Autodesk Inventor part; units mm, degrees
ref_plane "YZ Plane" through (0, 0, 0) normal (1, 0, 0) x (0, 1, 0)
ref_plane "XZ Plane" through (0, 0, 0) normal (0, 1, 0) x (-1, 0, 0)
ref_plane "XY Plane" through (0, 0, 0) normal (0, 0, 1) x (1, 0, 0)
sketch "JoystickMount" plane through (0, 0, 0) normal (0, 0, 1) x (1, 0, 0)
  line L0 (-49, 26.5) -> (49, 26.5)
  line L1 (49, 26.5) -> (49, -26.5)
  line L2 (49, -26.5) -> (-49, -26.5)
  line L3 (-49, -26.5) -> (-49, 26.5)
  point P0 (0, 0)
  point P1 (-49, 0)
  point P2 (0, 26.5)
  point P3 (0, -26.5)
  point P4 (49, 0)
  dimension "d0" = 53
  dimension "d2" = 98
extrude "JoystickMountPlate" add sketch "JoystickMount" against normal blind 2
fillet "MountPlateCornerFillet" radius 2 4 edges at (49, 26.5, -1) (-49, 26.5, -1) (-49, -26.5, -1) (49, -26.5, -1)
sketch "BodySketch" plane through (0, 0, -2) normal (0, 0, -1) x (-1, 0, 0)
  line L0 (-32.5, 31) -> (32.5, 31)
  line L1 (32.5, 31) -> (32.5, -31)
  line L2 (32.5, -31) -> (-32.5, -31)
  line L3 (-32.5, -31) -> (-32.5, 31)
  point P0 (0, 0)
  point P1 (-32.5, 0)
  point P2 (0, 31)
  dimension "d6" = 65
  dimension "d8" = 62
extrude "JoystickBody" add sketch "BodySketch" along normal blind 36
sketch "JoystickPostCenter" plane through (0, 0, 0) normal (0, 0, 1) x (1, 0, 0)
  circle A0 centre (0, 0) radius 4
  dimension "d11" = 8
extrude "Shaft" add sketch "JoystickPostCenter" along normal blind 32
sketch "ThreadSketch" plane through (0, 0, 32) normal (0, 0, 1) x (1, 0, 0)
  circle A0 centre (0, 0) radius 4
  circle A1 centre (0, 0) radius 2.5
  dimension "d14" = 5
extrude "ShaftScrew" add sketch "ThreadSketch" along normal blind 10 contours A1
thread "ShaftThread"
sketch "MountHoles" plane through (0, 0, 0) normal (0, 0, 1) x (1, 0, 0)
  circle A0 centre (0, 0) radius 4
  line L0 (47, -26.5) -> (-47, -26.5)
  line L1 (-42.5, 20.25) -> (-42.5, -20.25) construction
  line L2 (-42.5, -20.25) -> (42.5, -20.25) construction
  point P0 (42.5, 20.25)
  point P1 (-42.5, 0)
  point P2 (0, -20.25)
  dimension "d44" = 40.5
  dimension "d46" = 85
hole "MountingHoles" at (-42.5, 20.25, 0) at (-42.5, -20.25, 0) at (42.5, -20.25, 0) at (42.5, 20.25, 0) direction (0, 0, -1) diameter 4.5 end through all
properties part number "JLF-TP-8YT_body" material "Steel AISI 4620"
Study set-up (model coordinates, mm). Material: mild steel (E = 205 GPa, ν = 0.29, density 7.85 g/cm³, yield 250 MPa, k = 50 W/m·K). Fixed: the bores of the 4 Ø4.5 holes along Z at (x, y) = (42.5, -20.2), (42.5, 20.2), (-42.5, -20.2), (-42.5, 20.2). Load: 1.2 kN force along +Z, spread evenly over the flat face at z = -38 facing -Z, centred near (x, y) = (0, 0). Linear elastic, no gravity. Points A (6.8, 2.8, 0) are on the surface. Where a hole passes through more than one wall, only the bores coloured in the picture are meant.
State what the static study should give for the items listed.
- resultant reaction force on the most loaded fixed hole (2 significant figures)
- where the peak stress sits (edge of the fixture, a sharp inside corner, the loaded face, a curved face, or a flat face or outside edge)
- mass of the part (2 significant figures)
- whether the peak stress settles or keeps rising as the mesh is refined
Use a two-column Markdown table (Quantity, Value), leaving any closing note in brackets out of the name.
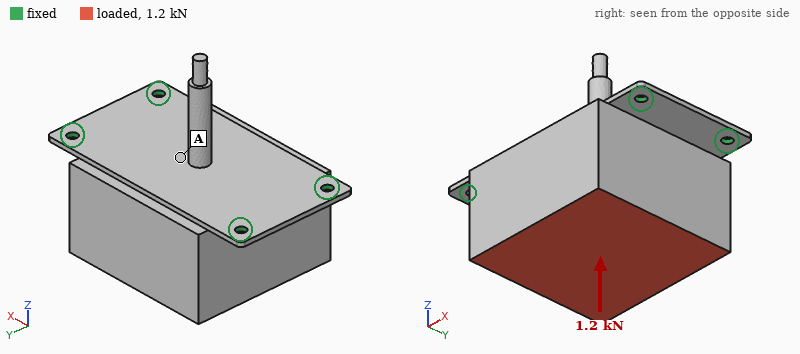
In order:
| Quantity | Value |
|---|---|
| resultant reaction force on the most loaded fixed hole | 350 N |
| where the peak stress sits | edge of the fixture |
| mass of the part | 1.2 kg |
| whether the peak stress settles or keeps rising as the mesh is refined | keeps rising |
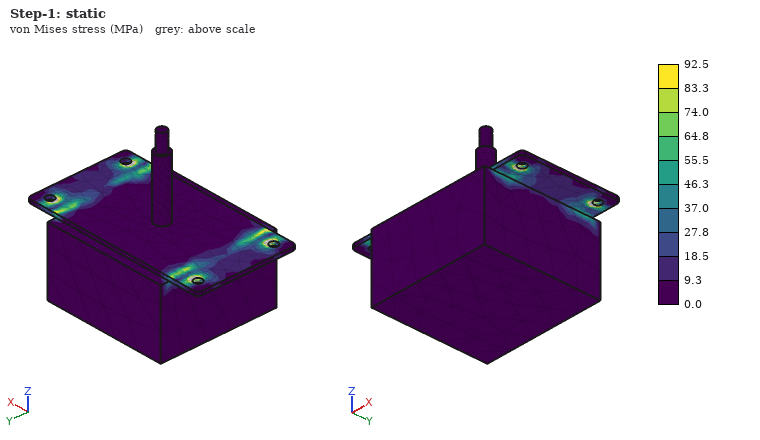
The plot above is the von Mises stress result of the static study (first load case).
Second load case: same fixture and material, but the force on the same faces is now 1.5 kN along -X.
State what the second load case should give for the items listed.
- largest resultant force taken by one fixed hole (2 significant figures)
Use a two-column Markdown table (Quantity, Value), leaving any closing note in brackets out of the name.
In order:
| Quantity | Value |
|---|---|
| largest resultant force taken by one fixed hole | 530 N |
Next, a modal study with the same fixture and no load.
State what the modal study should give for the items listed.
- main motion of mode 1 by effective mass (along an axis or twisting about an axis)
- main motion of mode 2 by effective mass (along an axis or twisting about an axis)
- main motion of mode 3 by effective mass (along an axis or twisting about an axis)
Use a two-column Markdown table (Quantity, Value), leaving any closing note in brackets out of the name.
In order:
| Quantity | Value |
|---|---|
| main motion of mode 1 by effective mass | along Y |
| main motion of mode 2 by effective mass | along Z |
| main motion of mode 3 by effective mass | along X |
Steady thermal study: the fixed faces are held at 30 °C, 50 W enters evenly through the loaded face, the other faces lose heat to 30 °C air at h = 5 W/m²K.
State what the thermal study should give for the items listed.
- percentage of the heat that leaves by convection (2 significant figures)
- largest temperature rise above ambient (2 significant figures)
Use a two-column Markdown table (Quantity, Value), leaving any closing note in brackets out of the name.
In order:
| Quantity | Value |
|---|---|
| percentage of the heat that leaves by convection | 12 % |
| largest temperature rise above ambient | 81 K |
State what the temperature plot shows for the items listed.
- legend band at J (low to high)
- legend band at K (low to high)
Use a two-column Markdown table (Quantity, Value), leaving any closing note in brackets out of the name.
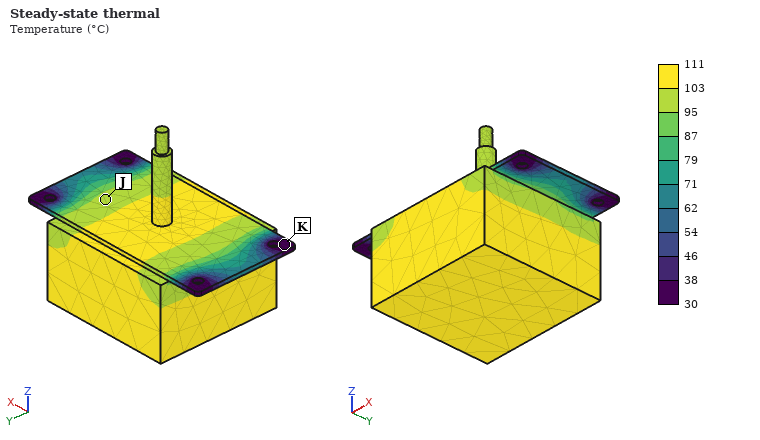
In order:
| Quantity | Value |
|---|---|
| legend band at J | 95 to 103 °C |
| legend band at K | 30 to 38 °C |
